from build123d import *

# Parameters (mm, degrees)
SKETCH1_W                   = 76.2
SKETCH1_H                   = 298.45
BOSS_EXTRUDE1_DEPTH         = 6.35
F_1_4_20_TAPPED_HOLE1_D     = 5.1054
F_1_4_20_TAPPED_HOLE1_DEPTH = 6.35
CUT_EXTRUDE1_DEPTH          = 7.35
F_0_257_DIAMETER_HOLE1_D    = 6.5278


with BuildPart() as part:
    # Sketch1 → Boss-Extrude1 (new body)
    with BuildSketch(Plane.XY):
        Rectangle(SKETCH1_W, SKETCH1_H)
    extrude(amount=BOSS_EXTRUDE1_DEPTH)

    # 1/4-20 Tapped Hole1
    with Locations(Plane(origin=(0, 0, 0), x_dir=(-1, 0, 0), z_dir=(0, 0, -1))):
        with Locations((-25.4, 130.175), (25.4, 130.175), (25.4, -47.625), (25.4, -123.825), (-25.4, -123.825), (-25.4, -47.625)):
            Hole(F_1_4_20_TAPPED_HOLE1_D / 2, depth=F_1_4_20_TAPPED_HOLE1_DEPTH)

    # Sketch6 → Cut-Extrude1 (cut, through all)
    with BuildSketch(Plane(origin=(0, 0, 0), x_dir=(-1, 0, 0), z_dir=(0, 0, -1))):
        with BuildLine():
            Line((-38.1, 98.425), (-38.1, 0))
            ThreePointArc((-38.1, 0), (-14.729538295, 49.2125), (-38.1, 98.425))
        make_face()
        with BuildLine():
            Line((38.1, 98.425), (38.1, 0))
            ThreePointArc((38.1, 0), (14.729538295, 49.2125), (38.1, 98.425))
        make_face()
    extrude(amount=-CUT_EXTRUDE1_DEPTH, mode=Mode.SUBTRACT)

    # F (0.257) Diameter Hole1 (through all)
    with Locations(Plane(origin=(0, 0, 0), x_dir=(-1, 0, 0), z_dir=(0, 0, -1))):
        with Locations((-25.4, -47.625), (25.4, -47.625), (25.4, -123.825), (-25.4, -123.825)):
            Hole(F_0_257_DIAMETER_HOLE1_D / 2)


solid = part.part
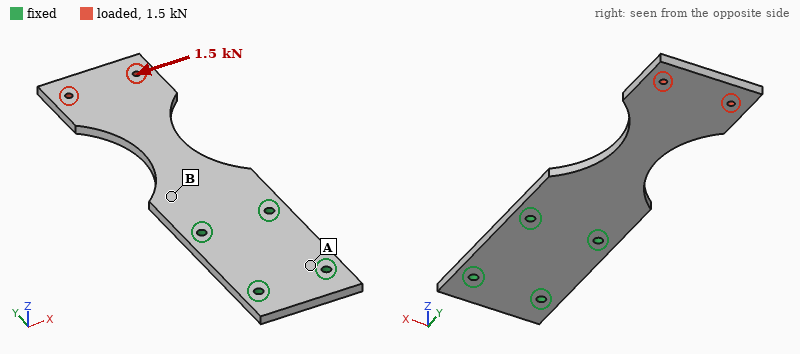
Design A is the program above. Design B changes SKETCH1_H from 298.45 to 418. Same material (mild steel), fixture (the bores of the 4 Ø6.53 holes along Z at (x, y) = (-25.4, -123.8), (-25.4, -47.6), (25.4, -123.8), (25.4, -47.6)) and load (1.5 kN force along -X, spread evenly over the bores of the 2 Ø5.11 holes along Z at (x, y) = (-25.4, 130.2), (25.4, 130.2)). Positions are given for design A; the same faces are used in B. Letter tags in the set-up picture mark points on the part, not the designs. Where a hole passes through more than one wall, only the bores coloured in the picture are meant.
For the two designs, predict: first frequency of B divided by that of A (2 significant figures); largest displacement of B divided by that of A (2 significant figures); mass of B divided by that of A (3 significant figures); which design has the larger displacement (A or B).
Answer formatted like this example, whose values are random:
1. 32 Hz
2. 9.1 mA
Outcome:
1. 0.55
2. 1.5
3. 1.47
4. B
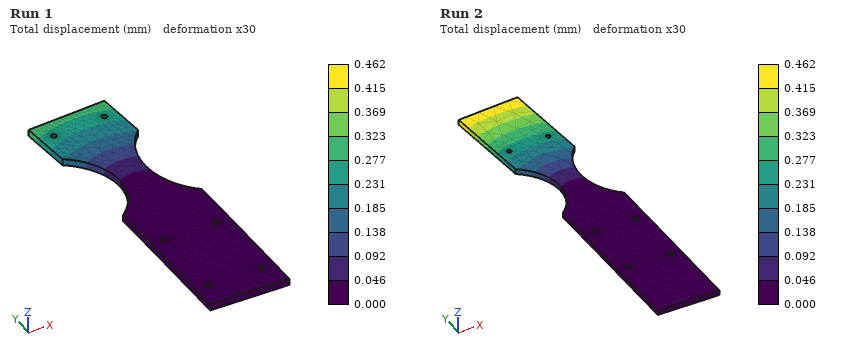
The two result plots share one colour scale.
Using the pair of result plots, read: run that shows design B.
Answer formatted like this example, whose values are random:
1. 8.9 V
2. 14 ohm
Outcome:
1. Run 2
